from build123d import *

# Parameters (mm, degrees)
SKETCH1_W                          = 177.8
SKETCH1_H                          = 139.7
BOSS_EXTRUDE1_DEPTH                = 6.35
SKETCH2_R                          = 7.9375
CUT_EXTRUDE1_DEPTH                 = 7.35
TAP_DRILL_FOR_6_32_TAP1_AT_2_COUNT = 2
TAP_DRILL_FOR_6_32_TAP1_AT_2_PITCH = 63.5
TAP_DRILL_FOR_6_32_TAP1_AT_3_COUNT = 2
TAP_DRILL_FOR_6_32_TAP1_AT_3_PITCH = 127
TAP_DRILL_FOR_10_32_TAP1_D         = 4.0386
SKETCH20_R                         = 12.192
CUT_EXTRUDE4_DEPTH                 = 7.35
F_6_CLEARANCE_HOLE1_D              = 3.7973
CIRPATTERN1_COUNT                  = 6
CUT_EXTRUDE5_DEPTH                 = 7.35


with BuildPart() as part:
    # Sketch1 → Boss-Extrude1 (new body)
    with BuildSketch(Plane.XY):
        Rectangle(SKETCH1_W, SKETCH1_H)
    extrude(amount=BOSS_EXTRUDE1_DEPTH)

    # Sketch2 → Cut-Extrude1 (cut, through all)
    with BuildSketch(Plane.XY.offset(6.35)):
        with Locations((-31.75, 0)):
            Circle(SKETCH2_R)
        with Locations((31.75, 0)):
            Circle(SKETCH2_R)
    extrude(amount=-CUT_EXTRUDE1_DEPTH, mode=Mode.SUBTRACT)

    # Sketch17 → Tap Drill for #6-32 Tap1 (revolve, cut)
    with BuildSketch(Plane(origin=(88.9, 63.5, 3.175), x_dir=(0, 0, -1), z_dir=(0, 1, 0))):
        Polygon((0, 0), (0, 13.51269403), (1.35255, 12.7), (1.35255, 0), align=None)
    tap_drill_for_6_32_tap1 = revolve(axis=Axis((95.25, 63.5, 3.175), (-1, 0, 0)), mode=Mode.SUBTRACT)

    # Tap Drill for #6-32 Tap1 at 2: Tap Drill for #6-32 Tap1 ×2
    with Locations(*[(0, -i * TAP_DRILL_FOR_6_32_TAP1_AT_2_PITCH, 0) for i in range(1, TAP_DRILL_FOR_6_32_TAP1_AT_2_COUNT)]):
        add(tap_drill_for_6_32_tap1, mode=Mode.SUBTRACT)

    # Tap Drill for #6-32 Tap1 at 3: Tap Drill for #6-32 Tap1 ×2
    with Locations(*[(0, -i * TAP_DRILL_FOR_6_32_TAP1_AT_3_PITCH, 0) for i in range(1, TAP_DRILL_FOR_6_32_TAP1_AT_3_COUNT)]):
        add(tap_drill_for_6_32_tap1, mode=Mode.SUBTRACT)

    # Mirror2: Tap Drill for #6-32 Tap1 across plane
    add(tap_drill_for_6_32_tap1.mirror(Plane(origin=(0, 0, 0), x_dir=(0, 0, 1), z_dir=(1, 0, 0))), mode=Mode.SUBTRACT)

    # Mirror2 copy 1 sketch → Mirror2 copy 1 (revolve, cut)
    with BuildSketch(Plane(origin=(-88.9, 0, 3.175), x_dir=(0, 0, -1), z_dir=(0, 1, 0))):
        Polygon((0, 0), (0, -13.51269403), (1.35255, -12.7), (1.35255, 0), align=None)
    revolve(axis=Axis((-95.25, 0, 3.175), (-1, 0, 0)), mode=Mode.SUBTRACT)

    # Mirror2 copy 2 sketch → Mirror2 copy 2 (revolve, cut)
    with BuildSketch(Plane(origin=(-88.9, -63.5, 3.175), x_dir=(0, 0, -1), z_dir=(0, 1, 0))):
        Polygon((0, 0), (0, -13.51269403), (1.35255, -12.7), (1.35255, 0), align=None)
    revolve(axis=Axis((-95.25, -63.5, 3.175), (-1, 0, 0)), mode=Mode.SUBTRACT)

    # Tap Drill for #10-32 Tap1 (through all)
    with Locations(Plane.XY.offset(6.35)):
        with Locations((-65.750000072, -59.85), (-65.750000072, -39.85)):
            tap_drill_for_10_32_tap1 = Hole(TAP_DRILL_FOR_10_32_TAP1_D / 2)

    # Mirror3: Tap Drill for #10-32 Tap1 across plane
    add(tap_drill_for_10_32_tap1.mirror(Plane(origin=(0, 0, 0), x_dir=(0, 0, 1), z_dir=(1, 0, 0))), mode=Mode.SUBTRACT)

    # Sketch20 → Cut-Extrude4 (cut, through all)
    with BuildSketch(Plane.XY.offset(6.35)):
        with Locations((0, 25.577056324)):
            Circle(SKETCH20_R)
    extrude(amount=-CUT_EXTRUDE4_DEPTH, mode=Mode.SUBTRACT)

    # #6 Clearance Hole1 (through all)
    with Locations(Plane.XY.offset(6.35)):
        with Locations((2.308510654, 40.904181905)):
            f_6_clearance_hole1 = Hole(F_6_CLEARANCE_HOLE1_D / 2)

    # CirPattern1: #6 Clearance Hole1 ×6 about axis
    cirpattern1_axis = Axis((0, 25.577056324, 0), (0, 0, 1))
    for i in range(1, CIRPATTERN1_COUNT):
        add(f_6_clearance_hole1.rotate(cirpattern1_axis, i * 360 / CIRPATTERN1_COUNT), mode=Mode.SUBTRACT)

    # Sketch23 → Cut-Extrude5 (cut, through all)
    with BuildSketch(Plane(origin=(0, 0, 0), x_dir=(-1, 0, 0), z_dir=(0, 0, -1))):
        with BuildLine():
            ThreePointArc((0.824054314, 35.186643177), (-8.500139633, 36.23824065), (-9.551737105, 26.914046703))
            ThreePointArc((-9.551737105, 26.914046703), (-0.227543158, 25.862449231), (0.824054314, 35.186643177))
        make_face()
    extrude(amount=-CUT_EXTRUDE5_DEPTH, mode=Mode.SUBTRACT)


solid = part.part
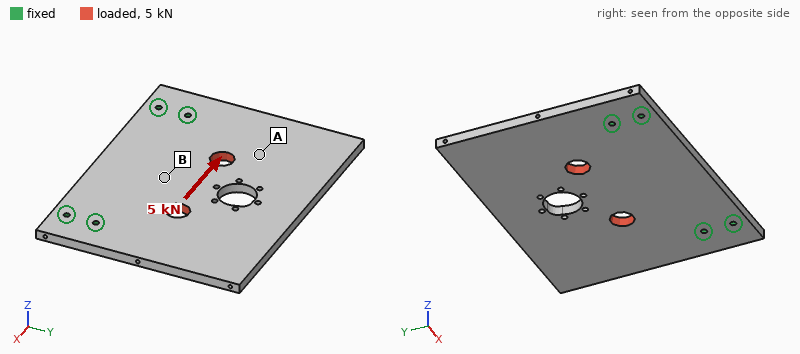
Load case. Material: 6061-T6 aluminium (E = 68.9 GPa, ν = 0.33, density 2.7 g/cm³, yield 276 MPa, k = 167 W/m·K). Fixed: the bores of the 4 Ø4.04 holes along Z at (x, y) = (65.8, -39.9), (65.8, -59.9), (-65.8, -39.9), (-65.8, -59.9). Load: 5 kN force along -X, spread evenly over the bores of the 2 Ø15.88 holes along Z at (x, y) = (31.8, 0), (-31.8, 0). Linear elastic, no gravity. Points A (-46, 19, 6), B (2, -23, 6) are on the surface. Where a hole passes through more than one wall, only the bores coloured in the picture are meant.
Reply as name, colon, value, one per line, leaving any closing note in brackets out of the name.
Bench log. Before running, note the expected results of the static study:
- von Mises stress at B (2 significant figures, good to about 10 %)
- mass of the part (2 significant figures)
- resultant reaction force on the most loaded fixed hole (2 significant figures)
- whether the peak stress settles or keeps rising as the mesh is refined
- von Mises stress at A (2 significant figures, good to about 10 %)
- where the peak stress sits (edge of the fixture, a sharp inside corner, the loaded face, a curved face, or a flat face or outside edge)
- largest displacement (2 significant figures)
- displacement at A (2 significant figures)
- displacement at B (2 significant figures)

von Mises stress at B: 8.1 MPa
mass of the part: 410 g
resultant reaction force on the most loaded fixed hole: 2.3 kN
whether the peak stress settles or keeps rising as the mesh is refined: keeps rising
von Mises stress at A: 2.2 MPa
where the peak stress sits: edge of the fixture
largest displacement: 17 µm
displacement at A: 14 µm
displacement at B: 7.7 µm
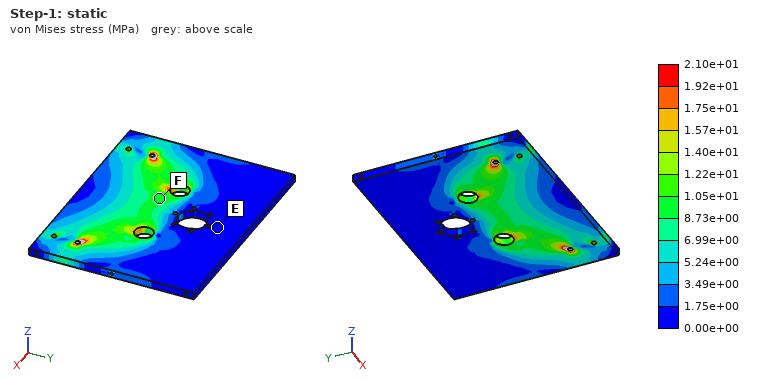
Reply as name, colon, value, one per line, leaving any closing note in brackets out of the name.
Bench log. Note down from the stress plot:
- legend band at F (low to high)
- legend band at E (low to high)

legend band at F: 8.73e+00 to 1.05e+01 MPa
legend band at E: 0.00e+00 to 1.75e+00 MPa
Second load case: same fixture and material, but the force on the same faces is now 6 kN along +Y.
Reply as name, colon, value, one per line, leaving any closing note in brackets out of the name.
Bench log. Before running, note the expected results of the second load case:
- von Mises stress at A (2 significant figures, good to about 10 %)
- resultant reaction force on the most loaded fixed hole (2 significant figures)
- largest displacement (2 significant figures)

von Mises stress at A: 5.7 MPa
resultant reaction force on the most loaded fixed hole: 2.0 kN
largest displacement: 13 µm
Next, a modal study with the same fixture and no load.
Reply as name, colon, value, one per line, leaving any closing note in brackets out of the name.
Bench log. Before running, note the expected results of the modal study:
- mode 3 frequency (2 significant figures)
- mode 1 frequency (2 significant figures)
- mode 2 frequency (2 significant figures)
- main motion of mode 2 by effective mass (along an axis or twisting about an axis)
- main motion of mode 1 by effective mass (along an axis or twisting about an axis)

mode 3 frequency: 1400 Hz
mode 1 frequency: 360 Hz
mode 2 frequency: 700 Hz
main motion of mode 2 by effective mass: twisting about Y
main motion of mode 1 by effective mass: along Z
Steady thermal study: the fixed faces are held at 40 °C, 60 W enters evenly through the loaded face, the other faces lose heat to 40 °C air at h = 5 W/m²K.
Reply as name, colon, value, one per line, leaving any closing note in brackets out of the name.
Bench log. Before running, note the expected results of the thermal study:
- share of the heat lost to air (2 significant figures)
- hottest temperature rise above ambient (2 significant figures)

share of the heat lost to air: 6.9 %
hottest temperature rise above ambient: 27 K
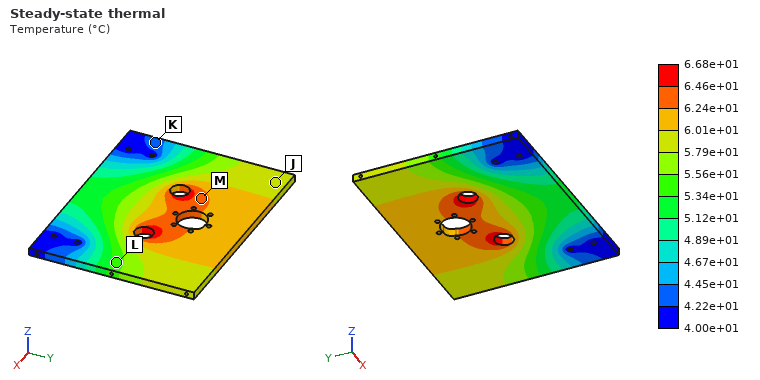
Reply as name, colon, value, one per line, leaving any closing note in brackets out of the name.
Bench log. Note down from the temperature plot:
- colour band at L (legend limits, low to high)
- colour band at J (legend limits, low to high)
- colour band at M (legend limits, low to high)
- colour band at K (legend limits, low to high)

colour band at L: 5.34e+01 to 5.56e+01 °C
colour band at J: 5.79e+01 to 6.01e+01 °C
colour band at M: 6.24e+01 to 6.46e+01 °C
colour band at K: 4.22e+01 to 4.45e+01 °C
